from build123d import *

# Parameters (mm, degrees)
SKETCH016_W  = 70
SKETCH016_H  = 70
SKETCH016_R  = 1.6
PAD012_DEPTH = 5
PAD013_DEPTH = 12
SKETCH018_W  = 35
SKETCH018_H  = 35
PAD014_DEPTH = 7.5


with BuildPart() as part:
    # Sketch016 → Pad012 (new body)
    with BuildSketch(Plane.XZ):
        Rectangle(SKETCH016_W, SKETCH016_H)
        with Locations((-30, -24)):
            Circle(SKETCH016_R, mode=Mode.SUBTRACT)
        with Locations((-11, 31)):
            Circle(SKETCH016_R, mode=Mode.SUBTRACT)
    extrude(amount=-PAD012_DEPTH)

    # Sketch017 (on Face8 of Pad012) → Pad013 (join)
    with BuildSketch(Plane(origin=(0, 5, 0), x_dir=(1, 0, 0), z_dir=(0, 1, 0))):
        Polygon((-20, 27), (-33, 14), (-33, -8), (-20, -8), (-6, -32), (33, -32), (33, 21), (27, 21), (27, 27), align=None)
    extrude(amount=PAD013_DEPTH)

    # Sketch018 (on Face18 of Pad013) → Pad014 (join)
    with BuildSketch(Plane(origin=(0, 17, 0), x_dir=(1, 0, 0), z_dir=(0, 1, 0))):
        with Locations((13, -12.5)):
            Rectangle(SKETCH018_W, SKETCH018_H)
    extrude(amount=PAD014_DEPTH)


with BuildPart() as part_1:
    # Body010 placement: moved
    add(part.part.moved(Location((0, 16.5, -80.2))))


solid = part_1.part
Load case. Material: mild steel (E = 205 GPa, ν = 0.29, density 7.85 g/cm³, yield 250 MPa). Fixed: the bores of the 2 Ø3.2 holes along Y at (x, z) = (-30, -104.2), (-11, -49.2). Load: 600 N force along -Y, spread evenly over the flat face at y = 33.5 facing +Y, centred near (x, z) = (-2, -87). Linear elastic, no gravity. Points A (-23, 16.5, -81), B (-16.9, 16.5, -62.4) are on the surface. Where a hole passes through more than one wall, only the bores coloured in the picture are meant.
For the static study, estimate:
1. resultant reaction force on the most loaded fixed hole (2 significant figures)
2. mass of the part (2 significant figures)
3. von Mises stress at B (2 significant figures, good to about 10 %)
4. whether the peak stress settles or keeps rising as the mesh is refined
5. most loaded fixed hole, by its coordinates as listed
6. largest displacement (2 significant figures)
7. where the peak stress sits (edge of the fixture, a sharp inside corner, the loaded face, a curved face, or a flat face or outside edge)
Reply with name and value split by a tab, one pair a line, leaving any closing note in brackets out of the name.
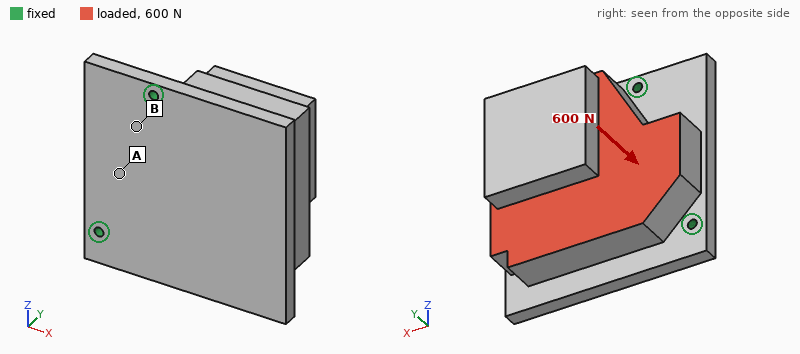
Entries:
resultant reaction force on the most loaded fixed hole	350 N
mass of the part	570 g
von Mises stress at B	15 MPa
whether the peak stress settles or keeps rising as the mesh is refined	keeps rising
most loaded fixed hole, by its coordinates as listed	(-30, -104.2)
largest displacement	55 µm
where the peak stress sits	edge of the fixture
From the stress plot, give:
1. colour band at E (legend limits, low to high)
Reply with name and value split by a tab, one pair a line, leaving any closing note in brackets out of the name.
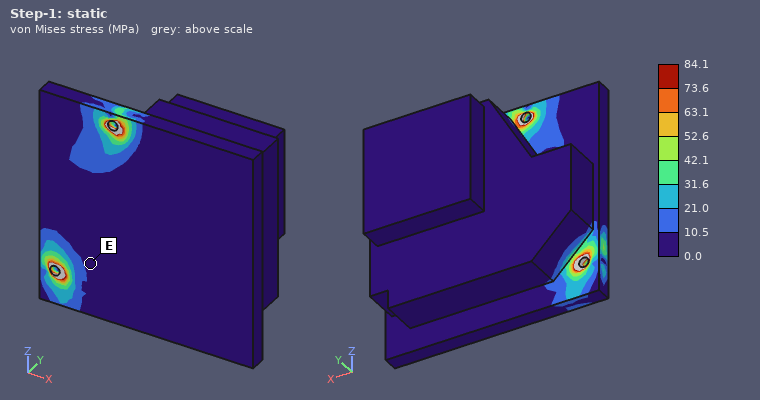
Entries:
colour band at E	0.0 to 10.5 MPa
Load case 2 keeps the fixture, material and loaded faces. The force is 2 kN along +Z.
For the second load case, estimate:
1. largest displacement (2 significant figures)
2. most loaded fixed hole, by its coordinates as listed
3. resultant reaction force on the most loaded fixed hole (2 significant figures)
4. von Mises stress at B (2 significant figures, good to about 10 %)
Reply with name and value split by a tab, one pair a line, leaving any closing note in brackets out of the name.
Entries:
largest displacement	46 µm
most loaded fixed hole, by its coordinates as listed	(-11, -49.2)
resultant reaction force on the most loaded fixed hole	1.4 kN
von Mises stress at B	14 MPa
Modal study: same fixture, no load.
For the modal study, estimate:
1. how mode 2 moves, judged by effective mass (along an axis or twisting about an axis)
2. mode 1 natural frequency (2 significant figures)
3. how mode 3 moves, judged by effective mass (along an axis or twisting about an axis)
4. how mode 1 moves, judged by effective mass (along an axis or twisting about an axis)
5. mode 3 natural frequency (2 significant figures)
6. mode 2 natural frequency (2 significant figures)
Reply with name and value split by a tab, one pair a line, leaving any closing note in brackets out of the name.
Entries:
how mode 2 moves, judged by effective mass	along Z
mode 1 natural frequency	840 Hz
how mode 3 moves, judged by effective mass	along Z
how mode 1 moves, judged by effective mass	along Y
mode 3 natural frequency	6400 Hz
mode 2 natural frequency	6100 Hz
